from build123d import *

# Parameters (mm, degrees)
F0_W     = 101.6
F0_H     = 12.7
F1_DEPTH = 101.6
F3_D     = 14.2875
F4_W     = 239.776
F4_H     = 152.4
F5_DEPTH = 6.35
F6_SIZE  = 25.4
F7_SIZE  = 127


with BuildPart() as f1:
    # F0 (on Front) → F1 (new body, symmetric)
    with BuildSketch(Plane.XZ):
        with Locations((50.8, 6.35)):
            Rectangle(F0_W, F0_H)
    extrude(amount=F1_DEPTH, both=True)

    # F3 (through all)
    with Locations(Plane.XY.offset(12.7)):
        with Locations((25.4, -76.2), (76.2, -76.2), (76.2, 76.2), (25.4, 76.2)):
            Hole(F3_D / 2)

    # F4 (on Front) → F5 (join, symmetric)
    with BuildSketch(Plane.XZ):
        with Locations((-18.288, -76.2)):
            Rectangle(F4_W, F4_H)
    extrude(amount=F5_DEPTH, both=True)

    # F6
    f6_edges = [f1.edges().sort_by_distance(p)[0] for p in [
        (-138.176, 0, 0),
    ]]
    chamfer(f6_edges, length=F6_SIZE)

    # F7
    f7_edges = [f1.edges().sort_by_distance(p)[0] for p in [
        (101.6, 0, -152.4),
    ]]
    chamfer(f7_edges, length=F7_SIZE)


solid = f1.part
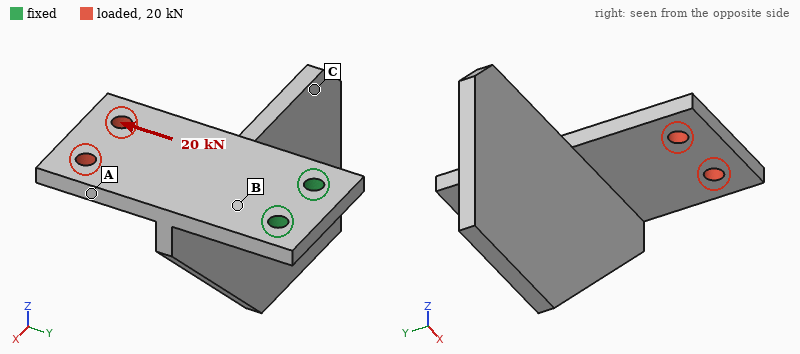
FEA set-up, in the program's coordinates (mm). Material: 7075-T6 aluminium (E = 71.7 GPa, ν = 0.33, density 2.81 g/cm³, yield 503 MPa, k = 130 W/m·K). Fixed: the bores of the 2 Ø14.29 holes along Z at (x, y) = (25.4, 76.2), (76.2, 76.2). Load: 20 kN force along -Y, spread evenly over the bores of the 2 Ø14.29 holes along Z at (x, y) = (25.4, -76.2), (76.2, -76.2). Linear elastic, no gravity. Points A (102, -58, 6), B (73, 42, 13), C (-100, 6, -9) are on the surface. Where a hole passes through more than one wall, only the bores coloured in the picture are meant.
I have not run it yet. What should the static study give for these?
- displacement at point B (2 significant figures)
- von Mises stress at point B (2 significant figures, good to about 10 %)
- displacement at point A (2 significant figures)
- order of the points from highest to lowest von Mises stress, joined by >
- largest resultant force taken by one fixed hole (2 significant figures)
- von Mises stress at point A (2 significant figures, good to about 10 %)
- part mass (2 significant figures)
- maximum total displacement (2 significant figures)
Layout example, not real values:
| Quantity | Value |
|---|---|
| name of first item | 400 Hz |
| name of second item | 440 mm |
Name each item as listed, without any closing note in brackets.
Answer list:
| Quantity | Value |
|---|---|
| displacement at point B | 8.3 µm |
| von Mises stress at point B | 18 MPa |
| displacement at point A | 30 µm |
| order of the points from highest to lowest von Mises stress, joined by > | B > A > C |
| largest resultant force taken by one fixed hole | 10 kN |
| von Mises stress at point A | 10 MPa |
| part mass | 1.7 kg |
| maximum total displacement | 41 µm |
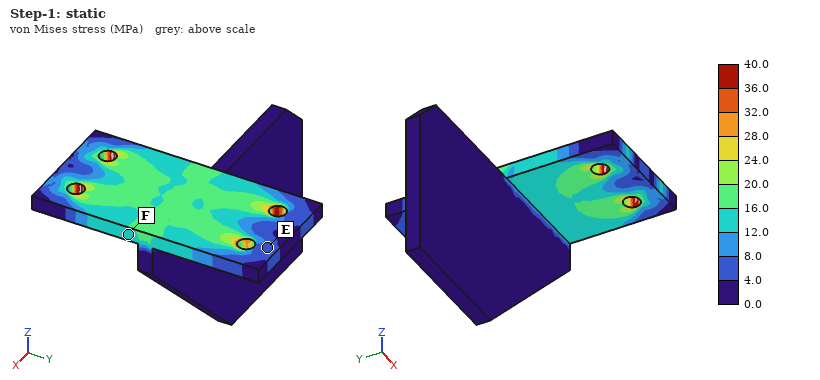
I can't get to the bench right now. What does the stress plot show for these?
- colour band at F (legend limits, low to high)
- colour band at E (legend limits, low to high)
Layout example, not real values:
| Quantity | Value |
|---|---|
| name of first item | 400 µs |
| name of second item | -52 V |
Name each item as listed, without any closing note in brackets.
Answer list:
| Quantity | Value |
|---|---|
| colour band at F | 12.0 to 16.0 MPa |
| colour band at E | 4.0 to 8.0 MPa |
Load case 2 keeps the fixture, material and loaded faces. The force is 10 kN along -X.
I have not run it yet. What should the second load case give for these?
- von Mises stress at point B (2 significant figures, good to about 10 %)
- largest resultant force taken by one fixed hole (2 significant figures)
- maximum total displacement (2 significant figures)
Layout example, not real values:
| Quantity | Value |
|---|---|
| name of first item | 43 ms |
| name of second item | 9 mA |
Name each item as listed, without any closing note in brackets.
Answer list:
| Quantity | Value |
|---|---|
| von Mises stress at point B | 35 MPa |
| largest resultant force taken by one fixed hole | 26 kN |
| maximum total displacement | 0.29 mm |
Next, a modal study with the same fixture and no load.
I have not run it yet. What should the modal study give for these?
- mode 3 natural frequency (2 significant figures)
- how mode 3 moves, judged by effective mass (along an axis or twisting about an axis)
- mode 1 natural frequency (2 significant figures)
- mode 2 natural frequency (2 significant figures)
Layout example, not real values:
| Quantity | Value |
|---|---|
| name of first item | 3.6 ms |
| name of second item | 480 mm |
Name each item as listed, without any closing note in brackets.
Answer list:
| Quantity | Value |
|---|---|
| mode 3 natural frequency | 370 Hz |
| how mode 3 moves, judged by effective mass | along Z |
| mode 1 natural frequency | 150 Hz |
| mode 2 natural frequency | 250 Hz |
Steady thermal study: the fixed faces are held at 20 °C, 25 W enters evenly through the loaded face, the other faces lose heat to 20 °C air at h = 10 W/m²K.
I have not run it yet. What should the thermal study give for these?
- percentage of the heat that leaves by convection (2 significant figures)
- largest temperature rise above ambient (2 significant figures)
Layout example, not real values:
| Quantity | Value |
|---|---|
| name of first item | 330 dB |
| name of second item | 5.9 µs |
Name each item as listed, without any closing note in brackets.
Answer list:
| Quantity | Value |
|---|---|
| percentage of the heat that leaves by convection | 32 % |
| largest temperature rise above ambient | 19 K |
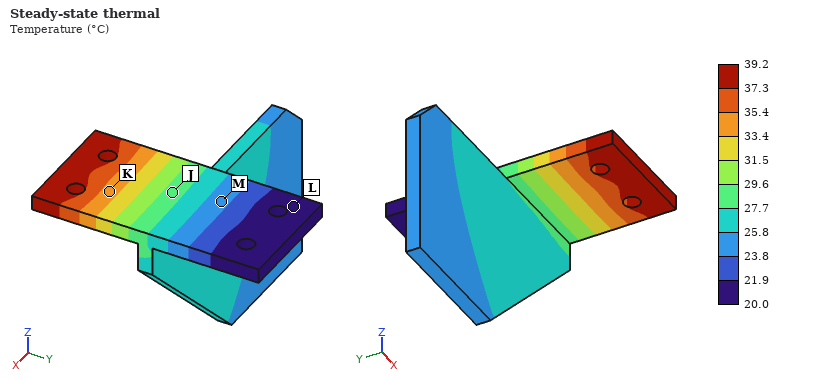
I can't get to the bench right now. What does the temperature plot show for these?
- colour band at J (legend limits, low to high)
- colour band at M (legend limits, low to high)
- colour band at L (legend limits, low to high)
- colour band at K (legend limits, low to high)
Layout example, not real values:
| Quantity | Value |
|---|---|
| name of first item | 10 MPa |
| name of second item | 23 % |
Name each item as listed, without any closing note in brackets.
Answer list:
| Quantity | Value |
|---|---|
| colour band at J | 27.7 to 29.6 °C |
| colour band at M | 23.8 to 25.8 °C |
| colour band at L | 20.0 to 21.9 °C |
| colour band at K | 33.4 to 35.4 °C |
